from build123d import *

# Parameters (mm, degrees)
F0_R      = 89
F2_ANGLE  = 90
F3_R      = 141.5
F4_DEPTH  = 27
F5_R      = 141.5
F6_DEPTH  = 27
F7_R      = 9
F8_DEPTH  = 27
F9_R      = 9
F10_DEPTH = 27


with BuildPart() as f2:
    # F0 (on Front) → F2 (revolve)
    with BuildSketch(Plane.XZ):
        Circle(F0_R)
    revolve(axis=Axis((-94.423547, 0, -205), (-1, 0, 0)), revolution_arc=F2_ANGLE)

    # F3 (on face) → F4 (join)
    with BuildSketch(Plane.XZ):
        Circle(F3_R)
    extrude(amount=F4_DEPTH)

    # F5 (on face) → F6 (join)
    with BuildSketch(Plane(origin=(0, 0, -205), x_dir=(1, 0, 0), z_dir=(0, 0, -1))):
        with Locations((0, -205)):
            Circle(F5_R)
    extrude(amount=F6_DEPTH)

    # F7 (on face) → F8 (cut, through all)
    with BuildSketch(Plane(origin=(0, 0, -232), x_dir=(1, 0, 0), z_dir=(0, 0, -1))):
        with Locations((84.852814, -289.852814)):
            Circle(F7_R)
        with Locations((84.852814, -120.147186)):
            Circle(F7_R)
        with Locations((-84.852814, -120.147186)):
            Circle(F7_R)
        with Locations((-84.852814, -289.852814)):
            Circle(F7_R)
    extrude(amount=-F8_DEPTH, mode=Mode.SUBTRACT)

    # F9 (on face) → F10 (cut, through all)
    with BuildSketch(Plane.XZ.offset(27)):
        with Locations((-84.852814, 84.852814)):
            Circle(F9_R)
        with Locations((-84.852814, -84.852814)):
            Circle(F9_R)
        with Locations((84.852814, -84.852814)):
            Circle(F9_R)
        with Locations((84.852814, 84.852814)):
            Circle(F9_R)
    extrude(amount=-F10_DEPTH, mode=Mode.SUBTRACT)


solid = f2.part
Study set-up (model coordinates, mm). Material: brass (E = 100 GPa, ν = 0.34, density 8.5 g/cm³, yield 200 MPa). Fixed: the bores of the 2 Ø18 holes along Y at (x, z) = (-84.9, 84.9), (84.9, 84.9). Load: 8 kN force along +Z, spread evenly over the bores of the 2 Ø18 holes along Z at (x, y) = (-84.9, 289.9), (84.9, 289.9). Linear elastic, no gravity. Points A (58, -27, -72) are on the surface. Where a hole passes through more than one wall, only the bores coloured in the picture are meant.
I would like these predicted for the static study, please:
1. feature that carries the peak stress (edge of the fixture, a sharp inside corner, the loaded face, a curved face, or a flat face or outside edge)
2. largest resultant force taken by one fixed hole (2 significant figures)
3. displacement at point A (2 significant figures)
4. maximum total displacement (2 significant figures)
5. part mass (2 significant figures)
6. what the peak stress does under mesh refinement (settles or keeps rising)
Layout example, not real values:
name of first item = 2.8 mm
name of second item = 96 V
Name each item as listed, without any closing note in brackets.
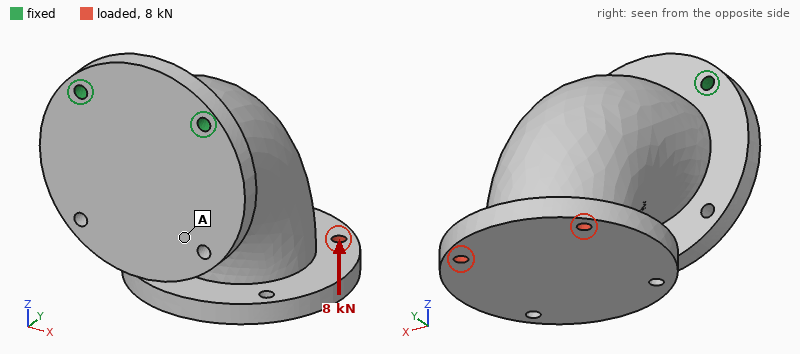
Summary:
feature that carries the peak stress = edge of the fixture
largest resultant force taken by one fixed hole = 4.1 kN
displacement at point A = 0.38 mm
maximum total displacement = 1.3 mm
part mass = 97 kg
what the peak stress does under mesh refinement = keeps rising
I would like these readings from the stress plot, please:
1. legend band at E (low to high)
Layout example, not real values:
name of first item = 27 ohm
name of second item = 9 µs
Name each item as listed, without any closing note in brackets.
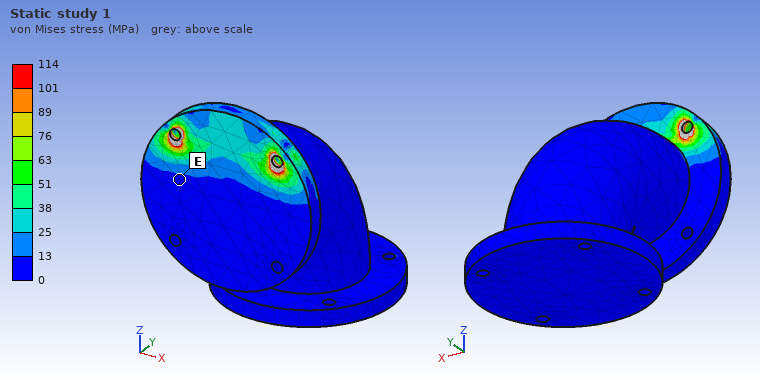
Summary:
legend band at E = 0 to 13 MPa
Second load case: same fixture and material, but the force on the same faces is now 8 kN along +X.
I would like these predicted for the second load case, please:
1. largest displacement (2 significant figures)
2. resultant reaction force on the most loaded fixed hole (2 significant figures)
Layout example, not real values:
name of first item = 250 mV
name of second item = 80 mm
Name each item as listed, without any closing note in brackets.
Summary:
largest displacement = 0.15 mm
resultant reaction force on the most loaded fixed hole = 21 kN
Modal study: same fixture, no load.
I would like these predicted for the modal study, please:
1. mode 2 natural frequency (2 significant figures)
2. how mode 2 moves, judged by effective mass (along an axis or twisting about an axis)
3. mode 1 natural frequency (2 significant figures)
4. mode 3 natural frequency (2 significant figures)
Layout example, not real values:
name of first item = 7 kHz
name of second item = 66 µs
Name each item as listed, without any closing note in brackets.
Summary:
mode 2 natural frequency = 240 Hz
how mode 2 moves, judged by effective mass = along X
mode 1 natural frequency = 64 Hz
mode 3 natural frequency = 710 Hz
